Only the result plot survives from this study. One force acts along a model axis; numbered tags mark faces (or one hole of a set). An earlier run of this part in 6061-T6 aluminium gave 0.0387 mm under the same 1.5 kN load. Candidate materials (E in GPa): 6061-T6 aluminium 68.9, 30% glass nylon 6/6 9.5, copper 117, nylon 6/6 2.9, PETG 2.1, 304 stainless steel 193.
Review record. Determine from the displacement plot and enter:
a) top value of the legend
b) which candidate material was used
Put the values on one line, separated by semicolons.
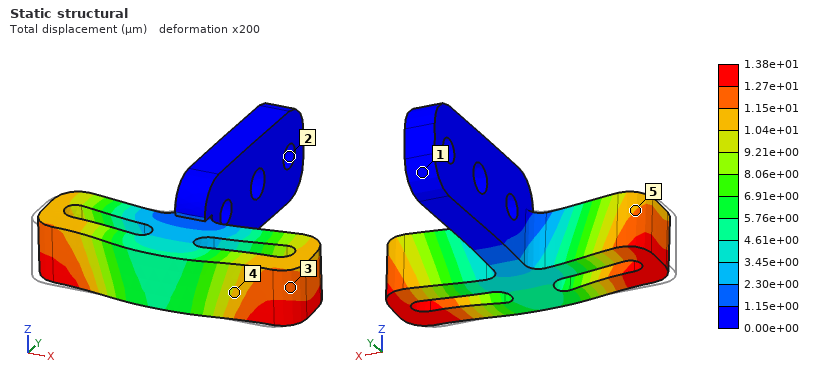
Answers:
1.38e+01 µm; 304 stainless steel
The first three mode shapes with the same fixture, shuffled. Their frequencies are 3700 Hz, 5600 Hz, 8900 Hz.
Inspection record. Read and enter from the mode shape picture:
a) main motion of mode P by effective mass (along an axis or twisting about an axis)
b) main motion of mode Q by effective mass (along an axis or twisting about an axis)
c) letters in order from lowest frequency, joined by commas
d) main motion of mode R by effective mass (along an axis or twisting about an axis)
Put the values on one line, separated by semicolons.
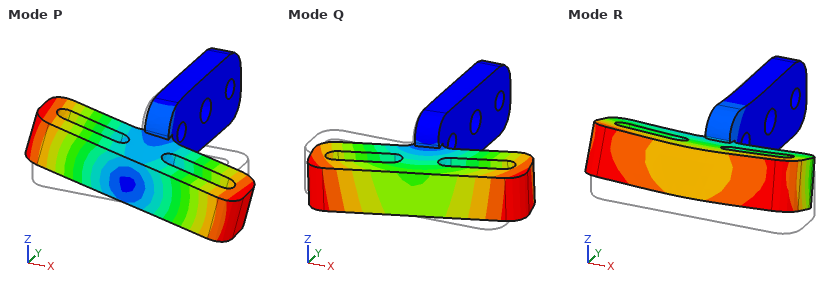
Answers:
twisting about Y; along X; Q, P, R; along Z
